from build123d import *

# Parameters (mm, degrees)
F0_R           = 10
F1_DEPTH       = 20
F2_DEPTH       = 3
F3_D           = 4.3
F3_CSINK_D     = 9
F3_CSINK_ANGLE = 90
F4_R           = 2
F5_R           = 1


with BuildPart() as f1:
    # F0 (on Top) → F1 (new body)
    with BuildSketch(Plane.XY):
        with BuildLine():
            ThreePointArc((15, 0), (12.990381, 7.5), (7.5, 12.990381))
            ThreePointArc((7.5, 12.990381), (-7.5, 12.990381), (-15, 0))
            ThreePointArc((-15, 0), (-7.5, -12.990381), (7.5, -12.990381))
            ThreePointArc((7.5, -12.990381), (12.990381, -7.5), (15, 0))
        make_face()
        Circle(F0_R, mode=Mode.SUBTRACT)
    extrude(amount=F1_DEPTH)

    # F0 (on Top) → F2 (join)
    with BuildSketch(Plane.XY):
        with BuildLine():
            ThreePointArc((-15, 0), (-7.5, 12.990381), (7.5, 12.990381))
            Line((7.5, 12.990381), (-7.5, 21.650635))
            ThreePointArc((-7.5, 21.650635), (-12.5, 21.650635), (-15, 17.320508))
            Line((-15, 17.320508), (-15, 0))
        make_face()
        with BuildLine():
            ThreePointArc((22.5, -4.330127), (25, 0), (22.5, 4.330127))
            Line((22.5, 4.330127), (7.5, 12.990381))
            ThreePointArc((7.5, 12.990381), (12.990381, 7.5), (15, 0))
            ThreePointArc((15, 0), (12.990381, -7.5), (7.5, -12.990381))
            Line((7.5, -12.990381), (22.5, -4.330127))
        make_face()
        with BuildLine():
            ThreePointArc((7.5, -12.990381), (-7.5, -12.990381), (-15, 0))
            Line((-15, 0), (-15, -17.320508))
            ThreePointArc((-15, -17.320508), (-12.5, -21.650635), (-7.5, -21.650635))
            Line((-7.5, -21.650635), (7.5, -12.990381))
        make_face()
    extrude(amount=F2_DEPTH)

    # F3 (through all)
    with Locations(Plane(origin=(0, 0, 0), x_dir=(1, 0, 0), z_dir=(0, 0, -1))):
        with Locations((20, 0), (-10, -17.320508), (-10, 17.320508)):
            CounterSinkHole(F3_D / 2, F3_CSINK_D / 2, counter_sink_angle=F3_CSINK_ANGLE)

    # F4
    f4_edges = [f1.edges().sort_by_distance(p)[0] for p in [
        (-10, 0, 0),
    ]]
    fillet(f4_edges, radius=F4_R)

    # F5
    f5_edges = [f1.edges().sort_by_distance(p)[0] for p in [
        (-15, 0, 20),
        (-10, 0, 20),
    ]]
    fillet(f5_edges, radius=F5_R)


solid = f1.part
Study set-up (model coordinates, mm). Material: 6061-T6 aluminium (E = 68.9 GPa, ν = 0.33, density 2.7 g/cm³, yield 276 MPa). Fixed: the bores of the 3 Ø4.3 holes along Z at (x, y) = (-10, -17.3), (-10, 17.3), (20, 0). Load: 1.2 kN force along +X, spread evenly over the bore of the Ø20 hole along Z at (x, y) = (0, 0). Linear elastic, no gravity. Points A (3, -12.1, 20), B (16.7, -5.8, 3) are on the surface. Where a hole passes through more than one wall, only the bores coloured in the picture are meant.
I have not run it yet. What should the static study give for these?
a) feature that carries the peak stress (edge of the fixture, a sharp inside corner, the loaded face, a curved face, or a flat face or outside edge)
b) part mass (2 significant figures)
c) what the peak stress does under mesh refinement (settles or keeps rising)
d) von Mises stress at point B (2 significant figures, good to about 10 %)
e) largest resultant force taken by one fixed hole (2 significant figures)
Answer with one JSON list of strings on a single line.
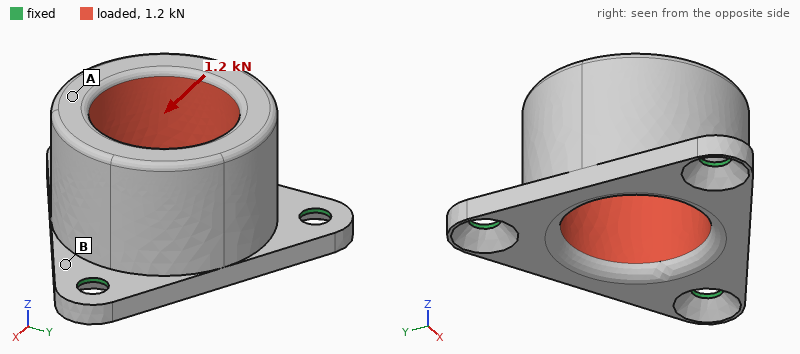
["edge of the fixture", "24 g", "keeps rising", "34 MPa", "500 N"]
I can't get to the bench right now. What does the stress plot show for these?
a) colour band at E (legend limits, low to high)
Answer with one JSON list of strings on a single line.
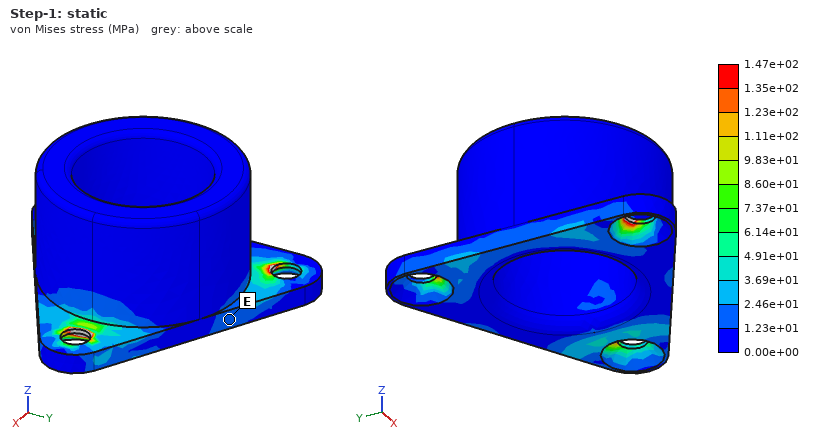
["1.23e+01 to 2.46e+01 MPa"]
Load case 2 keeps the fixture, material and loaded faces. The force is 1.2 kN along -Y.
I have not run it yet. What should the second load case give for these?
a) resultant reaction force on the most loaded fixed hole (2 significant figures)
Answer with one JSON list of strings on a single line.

["490 N"]
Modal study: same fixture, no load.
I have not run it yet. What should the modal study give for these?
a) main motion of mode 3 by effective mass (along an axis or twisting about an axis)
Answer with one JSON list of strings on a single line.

["along Z"]
